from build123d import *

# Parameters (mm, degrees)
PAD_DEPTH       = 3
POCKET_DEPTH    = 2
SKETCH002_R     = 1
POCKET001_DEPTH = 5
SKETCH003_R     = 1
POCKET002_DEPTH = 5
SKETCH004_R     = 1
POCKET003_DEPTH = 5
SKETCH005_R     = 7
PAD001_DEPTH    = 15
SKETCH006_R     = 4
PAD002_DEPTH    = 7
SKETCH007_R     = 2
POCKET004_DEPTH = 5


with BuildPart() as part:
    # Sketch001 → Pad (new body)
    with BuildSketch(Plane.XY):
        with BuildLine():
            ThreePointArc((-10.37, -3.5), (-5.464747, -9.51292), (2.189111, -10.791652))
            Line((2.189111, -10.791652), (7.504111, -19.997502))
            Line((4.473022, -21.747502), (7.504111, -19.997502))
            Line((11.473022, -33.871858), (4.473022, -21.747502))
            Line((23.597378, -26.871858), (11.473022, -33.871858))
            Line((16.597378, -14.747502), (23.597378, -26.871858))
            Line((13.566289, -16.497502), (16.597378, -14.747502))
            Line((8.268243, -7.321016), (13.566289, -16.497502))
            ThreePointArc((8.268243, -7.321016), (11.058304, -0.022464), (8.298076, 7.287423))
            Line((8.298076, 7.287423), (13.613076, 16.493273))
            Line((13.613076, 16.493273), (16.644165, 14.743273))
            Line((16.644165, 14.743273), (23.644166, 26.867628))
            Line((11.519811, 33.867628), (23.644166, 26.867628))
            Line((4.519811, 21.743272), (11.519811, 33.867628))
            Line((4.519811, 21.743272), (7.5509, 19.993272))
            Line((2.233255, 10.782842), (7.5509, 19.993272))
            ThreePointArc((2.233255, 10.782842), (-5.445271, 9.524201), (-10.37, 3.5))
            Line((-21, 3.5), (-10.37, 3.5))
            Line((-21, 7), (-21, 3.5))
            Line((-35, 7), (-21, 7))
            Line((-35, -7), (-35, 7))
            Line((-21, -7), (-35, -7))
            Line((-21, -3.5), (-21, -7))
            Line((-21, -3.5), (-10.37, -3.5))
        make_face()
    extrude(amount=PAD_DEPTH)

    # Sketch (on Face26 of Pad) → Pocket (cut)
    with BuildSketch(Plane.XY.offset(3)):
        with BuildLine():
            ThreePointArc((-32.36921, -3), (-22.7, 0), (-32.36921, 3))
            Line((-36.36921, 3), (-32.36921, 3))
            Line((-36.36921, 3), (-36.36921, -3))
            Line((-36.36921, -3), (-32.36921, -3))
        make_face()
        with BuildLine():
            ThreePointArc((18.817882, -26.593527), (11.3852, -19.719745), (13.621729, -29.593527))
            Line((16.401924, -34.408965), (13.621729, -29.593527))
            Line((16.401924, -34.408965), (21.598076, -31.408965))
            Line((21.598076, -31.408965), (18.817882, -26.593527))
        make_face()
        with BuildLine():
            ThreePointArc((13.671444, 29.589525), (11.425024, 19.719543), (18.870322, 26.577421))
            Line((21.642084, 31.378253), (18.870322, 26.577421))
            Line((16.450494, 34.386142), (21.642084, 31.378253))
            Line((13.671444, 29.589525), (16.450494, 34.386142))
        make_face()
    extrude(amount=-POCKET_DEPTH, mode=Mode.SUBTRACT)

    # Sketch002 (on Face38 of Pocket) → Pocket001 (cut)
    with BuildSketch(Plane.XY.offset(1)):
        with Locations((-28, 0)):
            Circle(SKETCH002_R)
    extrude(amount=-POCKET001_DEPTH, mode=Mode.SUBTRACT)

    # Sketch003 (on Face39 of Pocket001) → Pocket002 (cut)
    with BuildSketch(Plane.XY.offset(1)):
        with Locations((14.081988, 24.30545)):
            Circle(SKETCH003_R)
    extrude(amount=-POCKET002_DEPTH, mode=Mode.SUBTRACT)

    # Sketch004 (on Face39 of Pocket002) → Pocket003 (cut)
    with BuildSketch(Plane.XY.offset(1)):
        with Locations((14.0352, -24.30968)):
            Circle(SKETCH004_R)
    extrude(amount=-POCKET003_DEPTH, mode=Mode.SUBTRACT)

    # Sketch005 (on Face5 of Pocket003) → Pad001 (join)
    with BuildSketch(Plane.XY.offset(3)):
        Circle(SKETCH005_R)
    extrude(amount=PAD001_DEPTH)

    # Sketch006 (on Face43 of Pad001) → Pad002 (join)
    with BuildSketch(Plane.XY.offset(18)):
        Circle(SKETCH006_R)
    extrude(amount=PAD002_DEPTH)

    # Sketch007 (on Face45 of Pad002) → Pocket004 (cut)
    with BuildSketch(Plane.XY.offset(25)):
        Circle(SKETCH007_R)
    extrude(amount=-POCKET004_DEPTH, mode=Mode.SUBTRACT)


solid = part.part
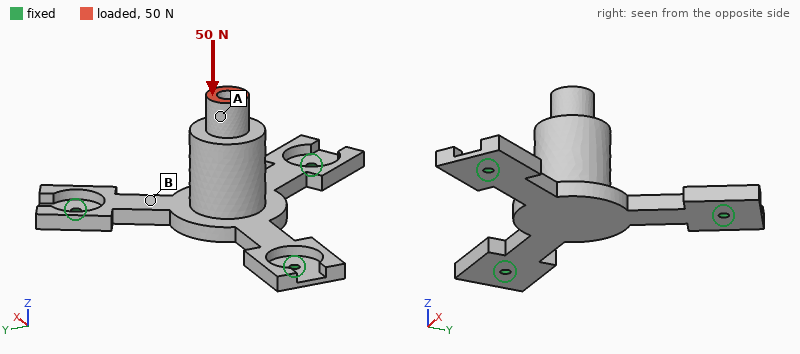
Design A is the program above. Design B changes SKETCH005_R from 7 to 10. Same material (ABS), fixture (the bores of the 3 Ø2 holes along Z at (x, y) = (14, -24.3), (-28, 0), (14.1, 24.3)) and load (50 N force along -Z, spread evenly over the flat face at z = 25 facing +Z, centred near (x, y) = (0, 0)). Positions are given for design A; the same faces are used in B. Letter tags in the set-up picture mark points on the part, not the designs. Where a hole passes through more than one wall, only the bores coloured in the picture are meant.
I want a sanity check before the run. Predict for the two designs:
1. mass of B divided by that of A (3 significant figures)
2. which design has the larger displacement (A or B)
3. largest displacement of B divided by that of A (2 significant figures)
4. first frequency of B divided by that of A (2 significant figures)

1.43
A
0.74
0.92
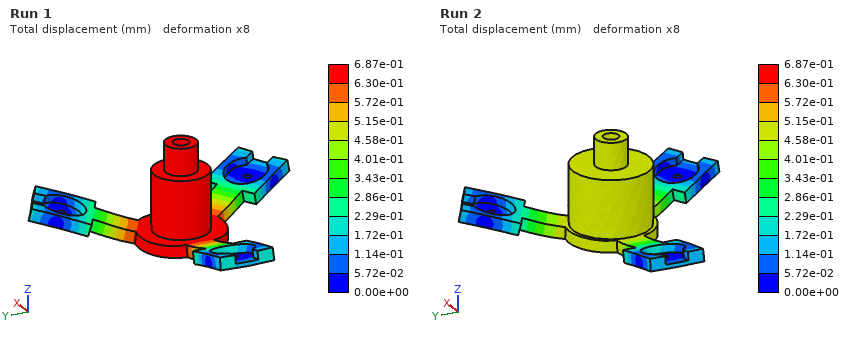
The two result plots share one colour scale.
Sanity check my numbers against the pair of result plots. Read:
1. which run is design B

Run 2
